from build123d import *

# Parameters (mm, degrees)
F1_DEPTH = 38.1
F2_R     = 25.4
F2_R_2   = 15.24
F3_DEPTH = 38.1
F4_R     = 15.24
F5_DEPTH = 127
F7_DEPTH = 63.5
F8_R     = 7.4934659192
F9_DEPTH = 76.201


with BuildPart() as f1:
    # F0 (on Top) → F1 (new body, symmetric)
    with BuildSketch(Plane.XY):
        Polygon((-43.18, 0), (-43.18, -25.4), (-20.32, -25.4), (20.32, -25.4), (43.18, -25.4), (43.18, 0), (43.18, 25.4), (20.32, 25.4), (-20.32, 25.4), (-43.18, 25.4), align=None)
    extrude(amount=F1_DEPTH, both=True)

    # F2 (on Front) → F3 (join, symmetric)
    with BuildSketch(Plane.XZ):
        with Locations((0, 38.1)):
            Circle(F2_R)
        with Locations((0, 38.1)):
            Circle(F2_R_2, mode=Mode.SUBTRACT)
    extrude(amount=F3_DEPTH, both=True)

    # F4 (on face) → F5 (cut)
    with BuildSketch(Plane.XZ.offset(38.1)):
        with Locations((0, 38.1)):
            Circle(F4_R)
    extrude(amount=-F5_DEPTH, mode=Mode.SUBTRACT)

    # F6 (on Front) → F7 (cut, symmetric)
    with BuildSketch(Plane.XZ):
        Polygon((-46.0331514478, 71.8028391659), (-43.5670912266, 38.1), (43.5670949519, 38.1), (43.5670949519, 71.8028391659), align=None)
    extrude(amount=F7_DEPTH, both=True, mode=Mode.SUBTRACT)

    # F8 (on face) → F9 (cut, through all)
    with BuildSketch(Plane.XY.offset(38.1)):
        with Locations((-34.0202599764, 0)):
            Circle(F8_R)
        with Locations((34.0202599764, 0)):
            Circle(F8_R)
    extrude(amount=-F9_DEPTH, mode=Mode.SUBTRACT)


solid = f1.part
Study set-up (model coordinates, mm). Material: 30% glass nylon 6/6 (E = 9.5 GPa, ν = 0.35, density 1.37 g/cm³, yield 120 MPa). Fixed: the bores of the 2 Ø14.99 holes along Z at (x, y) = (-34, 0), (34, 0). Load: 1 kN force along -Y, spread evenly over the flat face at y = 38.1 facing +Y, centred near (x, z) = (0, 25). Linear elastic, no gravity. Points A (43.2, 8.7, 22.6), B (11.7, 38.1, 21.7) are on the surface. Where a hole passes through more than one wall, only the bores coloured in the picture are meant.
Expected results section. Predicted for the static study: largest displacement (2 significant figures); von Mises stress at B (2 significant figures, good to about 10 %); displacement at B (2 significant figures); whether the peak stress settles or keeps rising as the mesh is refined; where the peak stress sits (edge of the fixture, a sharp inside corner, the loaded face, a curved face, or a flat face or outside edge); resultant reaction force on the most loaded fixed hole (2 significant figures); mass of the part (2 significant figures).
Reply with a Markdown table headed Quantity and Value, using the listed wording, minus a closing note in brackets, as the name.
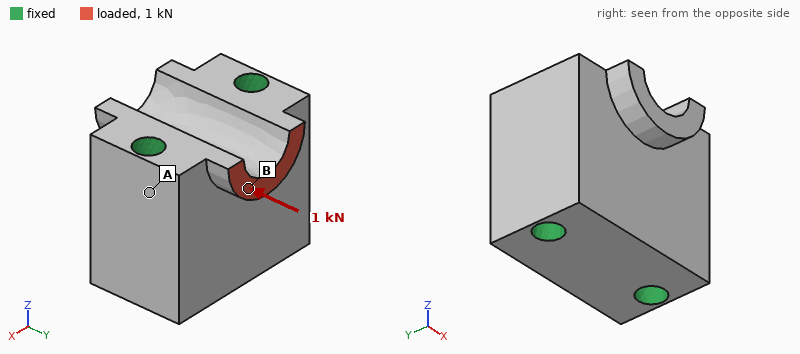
| Quantity | Value |
|---|---|
| largest displacement | 7.5 µm |
| von Mises stress at B | 1.4 MPa |
| displacement at B | 5.1 µm |
| whether the peak stress settles or keeps rising as the mesh is refined | keeps rising |
| where the peak stress sits | a sharp inside corner |
| resultant reaction force on the most loaded fixed hole | 520 N |
| mass of the part | 420 g |
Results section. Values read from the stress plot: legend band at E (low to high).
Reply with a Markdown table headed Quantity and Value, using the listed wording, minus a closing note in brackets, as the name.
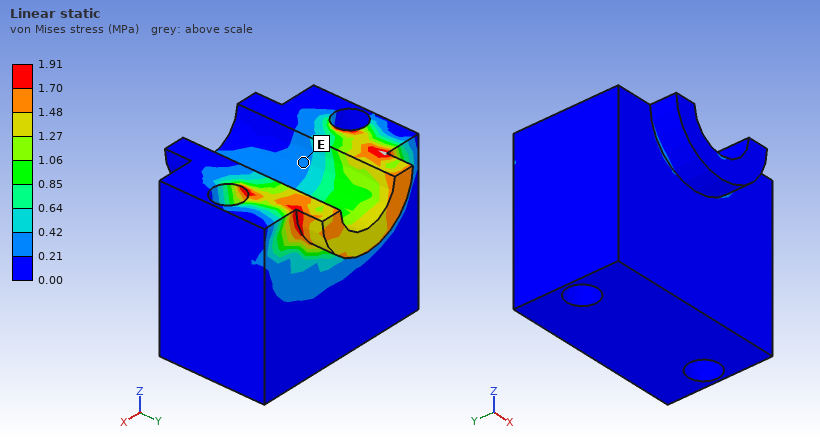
| Quantity | Value |
|---|---|
| legend band at E | 0.21 to 0.42 MPa |
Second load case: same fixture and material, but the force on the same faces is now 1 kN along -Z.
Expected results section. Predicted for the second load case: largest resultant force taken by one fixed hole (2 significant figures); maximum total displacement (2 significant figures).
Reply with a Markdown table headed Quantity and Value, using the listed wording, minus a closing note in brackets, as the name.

| Quantity | Value |
|---|---|
| largest resultant force taken by one fixed hole | 500 N |
| maximum total displacement | 35 µm |
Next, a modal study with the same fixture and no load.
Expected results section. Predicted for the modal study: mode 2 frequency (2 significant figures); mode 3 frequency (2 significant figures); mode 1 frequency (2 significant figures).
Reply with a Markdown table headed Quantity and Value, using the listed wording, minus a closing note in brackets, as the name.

| Quantity | Value |
|---|---|
| mode 2 frequency | 10 kHz |
| mode 3 frequency | 10 kHz |
| mode 1 frequency | 10 kHz |
